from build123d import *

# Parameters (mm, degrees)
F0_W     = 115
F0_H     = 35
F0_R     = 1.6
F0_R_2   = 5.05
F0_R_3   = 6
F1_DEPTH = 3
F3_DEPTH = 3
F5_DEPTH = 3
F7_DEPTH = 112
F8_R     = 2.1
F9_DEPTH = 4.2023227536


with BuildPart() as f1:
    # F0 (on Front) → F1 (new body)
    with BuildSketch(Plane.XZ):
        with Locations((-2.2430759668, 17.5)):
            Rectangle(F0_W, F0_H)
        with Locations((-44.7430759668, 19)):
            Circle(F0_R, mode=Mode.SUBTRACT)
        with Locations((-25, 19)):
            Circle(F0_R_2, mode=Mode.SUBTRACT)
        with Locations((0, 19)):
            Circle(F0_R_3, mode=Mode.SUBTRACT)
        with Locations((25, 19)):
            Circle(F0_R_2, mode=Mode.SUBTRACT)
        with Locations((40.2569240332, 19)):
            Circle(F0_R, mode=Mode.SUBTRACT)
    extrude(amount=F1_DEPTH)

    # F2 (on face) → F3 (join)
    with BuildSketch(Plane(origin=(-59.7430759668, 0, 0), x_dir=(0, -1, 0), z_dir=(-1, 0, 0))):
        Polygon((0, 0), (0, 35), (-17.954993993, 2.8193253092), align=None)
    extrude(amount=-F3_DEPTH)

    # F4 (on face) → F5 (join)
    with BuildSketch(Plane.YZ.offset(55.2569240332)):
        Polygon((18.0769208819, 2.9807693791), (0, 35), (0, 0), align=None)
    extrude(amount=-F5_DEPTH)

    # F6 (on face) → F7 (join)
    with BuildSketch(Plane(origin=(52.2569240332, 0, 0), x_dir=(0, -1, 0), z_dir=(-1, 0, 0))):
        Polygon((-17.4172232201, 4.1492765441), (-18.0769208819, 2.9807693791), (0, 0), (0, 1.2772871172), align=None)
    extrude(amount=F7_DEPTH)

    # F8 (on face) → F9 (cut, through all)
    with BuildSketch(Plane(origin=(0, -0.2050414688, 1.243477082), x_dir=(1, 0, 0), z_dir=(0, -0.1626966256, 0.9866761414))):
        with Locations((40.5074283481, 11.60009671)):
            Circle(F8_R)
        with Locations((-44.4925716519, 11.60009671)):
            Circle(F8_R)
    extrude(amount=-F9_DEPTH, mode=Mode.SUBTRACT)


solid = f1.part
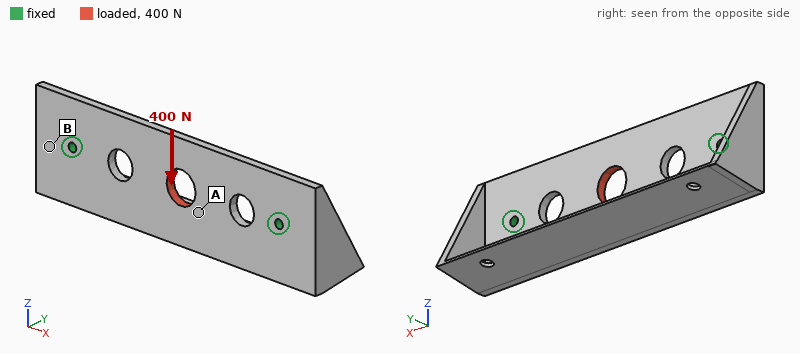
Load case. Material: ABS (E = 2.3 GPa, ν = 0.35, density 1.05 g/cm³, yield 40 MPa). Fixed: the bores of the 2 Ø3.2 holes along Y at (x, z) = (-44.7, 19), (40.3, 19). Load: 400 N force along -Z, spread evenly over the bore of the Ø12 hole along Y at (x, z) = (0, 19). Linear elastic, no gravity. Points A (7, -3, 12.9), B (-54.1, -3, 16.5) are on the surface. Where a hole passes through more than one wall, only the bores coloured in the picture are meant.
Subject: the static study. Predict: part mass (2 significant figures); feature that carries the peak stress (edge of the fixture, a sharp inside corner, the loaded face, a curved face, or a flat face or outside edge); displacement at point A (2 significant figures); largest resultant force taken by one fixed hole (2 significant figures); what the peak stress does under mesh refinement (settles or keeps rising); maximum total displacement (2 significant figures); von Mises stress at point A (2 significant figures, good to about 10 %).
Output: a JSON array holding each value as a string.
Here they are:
["16 g", "edge of the fixture", "0.30 mm", "220 N", "keeps rising", "0.42 mm", "4.8 MPa"]
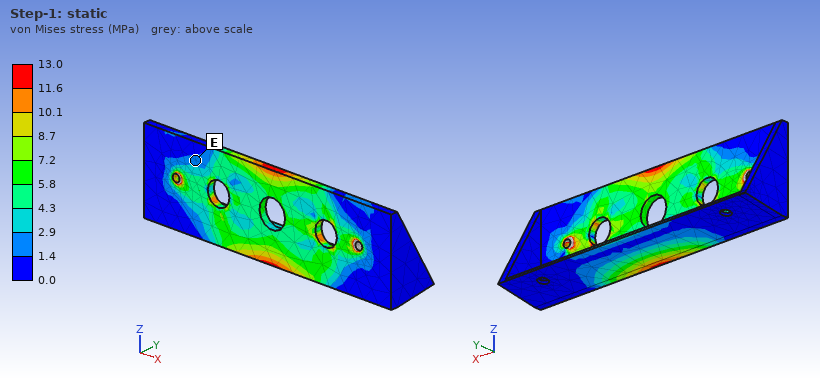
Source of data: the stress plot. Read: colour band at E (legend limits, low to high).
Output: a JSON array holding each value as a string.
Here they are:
["1.4 to 2.9 MPa"]
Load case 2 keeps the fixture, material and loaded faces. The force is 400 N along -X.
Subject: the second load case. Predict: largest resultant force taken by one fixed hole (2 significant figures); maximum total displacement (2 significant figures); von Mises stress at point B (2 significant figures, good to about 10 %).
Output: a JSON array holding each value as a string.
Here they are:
["200 N", "68 µm", "1.3 MPa"]
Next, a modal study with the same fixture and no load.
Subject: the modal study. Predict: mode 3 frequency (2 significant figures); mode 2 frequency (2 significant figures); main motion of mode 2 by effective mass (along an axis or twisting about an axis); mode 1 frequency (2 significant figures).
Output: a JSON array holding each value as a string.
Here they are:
["920 Hz", "740 Hz", "along Y", "660 Hz"]
